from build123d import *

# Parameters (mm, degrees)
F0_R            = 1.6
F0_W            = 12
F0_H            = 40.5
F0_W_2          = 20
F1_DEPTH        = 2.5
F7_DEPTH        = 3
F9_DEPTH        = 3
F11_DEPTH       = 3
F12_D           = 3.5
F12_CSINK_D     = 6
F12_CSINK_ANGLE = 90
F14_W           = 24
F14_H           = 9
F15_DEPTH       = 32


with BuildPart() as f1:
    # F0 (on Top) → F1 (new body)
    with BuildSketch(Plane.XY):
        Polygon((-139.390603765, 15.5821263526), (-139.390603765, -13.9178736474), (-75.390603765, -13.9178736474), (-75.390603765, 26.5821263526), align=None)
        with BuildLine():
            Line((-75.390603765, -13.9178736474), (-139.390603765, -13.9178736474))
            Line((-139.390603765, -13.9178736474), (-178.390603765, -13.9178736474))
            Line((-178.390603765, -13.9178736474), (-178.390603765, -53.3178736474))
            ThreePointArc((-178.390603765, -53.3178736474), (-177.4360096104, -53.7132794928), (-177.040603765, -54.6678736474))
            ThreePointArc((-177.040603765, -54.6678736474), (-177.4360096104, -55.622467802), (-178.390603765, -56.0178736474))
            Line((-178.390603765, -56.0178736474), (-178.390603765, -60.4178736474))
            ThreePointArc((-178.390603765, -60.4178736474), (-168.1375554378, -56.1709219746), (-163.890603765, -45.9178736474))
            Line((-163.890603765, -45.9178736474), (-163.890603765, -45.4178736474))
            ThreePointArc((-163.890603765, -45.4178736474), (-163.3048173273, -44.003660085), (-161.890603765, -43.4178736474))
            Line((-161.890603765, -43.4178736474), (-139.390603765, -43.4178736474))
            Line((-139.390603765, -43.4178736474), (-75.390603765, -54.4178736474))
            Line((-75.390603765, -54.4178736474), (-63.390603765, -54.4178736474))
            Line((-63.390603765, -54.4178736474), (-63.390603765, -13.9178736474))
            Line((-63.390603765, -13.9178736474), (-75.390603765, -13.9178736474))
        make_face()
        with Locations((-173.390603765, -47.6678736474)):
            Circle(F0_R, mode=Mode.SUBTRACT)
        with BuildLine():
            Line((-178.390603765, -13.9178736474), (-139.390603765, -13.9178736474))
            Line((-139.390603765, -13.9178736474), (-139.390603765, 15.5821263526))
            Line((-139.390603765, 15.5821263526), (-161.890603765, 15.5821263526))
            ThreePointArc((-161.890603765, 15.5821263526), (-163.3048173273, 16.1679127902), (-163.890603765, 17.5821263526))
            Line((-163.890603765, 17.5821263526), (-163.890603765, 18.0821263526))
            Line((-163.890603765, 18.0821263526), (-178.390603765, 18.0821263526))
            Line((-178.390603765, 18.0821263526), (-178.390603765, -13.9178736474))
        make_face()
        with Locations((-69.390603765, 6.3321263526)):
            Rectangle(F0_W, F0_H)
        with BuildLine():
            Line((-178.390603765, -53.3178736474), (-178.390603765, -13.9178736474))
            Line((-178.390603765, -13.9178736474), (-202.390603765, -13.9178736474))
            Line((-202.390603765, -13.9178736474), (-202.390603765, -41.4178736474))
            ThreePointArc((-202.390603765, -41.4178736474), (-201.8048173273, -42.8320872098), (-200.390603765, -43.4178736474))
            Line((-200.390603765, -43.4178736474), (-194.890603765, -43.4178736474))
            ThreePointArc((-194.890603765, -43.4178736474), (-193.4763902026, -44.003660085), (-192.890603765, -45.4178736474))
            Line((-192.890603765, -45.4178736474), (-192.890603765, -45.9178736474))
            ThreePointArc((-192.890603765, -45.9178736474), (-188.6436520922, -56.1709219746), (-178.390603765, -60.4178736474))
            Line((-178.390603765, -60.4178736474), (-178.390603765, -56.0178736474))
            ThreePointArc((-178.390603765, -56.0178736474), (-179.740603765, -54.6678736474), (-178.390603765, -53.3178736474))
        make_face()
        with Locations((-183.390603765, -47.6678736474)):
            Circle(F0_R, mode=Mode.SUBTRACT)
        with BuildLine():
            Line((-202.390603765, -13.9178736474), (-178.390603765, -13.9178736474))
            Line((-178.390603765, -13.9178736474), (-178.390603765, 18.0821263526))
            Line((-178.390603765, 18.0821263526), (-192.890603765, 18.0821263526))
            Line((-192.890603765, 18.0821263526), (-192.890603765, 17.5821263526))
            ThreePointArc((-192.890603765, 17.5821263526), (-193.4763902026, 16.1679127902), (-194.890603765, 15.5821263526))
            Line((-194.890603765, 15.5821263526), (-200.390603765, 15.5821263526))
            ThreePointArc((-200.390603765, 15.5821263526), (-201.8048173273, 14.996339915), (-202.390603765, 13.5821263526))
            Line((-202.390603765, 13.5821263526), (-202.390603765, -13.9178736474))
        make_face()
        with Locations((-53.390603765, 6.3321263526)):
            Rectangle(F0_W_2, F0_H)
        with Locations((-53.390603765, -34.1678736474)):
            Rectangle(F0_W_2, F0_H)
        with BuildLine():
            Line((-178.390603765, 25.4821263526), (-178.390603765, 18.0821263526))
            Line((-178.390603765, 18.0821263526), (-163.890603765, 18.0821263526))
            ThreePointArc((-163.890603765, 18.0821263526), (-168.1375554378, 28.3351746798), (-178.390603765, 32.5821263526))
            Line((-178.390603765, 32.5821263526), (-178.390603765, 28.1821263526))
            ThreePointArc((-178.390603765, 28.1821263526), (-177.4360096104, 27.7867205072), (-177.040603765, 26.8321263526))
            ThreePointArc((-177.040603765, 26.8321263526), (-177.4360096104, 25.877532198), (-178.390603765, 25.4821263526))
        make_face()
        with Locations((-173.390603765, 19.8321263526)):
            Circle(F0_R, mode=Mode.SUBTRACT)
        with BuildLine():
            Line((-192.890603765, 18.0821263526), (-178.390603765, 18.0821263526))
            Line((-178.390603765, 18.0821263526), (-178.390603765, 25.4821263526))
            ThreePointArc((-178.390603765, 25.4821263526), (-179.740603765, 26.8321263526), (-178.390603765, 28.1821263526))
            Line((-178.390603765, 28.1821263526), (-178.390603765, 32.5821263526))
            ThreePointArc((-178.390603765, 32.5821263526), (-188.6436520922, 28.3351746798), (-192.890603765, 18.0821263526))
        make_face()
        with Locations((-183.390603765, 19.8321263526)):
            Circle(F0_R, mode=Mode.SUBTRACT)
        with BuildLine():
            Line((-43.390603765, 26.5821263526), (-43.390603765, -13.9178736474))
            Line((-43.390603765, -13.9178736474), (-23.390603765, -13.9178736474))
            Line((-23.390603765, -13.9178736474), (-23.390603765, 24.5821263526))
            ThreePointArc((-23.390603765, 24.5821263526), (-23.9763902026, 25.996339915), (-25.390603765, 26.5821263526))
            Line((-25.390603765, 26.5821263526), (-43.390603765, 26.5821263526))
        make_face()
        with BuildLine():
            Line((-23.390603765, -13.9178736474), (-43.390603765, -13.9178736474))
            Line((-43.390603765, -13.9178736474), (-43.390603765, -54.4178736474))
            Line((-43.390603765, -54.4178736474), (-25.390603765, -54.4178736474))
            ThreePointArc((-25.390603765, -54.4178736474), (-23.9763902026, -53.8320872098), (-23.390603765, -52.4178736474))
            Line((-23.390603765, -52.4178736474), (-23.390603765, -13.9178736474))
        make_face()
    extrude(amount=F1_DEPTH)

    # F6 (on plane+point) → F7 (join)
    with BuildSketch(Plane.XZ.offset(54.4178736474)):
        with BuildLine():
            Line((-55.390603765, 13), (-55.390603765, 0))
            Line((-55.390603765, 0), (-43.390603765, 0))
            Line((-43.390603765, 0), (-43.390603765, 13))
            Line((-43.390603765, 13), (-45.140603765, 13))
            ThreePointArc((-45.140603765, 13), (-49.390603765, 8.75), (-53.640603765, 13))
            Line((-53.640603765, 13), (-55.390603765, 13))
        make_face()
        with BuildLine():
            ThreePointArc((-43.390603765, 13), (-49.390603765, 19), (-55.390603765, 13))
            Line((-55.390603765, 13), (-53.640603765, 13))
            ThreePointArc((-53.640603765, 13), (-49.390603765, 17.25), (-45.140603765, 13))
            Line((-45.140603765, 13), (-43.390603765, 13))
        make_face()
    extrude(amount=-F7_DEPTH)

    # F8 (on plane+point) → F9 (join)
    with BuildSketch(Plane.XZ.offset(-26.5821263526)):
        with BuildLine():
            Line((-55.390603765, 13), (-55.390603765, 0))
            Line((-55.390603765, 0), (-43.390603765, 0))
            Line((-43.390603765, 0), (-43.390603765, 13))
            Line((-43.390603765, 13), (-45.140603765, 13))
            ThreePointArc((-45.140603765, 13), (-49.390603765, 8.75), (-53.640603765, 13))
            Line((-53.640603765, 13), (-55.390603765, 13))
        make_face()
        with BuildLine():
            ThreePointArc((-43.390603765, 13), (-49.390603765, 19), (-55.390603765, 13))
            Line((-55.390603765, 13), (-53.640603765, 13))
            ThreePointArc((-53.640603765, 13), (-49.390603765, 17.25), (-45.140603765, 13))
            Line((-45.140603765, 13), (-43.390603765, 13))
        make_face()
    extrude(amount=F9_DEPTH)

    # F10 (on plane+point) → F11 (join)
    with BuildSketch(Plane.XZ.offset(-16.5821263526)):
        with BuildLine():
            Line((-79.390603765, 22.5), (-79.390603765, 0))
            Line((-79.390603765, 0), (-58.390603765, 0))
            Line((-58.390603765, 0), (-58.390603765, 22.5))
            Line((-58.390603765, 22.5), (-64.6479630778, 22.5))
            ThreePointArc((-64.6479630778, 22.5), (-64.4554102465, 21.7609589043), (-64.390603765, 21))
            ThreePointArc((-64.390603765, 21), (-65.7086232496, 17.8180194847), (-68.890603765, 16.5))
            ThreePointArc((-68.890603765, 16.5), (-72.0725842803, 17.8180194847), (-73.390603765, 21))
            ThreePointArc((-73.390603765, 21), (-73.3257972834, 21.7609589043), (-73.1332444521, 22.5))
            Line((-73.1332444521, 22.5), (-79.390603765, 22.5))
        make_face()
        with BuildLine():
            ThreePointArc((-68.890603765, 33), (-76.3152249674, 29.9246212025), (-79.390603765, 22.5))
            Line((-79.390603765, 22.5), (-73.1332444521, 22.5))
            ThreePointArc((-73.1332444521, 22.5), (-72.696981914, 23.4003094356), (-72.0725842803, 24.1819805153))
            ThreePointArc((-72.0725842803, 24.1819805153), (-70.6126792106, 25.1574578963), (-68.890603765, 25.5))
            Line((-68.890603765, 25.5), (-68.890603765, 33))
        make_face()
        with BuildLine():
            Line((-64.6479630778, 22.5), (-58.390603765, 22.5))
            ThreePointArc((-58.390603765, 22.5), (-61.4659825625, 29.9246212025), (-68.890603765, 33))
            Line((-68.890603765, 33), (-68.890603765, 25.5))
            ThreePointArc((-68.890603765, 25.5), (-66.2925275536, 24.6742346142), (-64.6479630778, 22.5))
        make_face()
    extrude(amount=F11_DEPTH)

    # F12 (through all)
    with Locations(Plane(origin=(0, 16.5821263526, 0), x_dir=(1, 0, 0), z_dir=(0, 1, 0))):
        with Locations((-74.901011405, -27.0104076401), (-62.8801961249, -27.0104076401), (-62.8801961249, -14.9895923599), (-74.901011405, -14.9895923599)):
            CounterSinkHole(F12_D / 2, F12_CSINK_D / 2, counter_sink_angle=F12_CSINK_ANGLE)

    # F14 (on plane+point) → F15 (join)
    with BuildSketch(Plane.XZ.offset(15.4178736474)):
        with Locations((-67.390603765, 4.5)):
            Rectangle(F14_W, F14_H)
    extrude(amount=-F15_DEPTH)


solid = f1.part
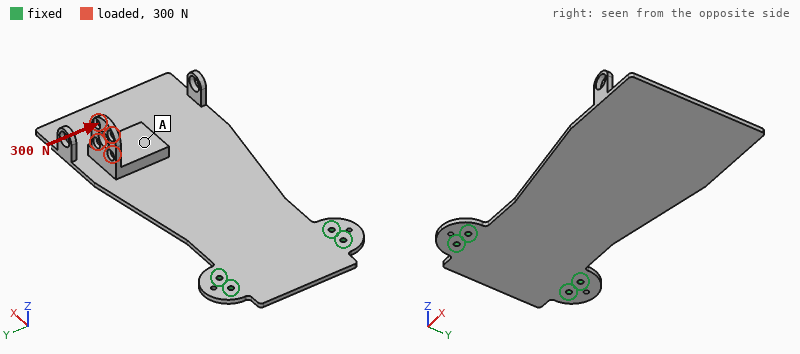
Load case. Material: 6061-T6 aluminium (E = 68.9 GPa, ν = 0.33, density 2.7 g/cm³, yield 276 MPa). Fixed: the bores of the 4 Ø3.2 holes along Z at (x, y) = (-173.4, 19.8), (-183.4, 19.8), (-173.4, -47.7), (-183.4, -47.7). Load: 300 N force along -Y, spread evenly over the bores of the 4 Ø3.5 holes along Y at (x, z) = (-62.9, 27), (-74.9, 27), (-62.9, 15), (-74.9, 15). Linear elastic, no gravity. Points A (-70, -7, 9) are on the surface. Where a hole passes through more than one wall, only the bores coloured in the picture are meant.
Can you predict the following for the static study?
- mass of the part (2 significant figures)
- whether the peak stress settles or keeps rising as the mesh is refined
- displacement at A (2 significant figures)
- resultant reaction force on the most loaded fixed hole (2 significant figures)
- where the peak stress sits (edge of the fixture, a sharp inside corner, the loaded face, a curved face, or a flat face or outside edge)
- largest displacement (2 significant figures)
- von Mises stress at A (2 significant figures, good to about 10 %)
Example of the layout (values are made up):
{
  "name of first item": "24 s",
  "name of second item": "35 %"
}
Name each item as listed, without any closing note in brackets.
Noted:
{
  "mass of the part": "110 g",
  "whether the peak stress settles or keeps rising as the mesh is refined": "keeps rising",
  "displacement at A": "0.49 mm",
  "resultant reaction force on the most loaded fixed hole": "370 N",
  "where the peak stress sits": "edge of the fixture",
  "largest displacement": "2.4 mm",
  "von Mises stress at A": "14 MPa"
}
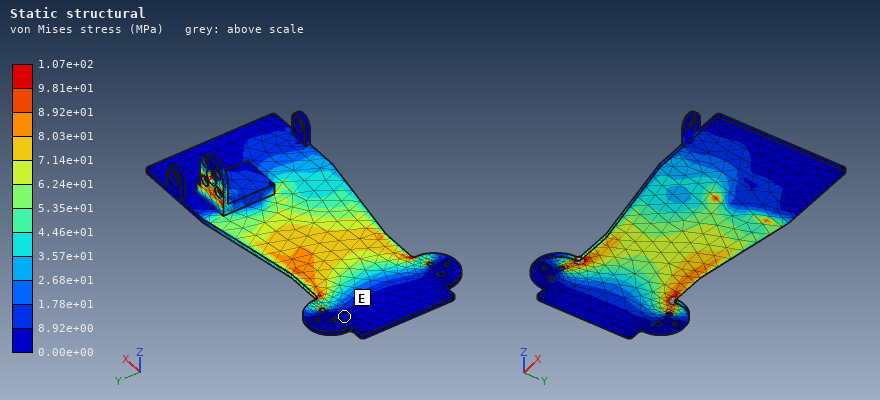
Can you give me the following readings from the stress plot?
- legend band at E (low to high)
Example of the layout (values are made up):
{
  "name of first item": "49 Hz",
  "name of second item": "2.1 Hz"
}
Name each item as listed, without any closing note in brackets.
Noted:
{
  "legend band at E": "0.00e+00 to 8.92e+00 MPa"
}
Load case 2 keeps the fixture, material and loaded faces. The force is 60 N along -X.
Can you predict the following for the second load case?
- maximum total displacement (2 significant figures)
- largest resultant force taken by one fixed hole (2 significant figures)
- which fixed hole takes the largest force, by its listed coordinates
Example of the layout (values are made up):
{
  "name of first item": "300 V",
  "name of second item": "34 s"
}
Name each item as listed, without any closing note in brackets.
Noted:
{
  "maximum total displacement": "2.2 mm",
  "largest resultant force taken by one fixed hole": "47 N",
  "which fixed hole takes the largest force, by its listed coordinates": "(-173.4, 19.8)"
}
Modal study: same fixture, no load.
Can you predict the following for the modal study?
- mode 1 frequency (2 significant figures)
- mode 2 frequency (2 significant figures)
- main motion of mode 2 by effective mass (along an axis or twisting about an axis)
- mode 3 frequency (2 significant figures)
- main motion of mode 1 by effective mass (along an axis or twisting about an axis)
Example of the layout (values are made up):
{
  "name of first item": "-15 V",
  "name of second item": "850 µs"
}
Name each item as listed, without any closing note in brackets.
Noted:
{
  "mode 1 frequency": "64 Hz",
  "mode 2 frequency": "300 Hz",
  "main motion of mode 2 by effective mass": "twisting about X",
  "mode 3 frequency": "530 Hz",
  "main motion of mode 1 by effective mass": "along Z"
}
